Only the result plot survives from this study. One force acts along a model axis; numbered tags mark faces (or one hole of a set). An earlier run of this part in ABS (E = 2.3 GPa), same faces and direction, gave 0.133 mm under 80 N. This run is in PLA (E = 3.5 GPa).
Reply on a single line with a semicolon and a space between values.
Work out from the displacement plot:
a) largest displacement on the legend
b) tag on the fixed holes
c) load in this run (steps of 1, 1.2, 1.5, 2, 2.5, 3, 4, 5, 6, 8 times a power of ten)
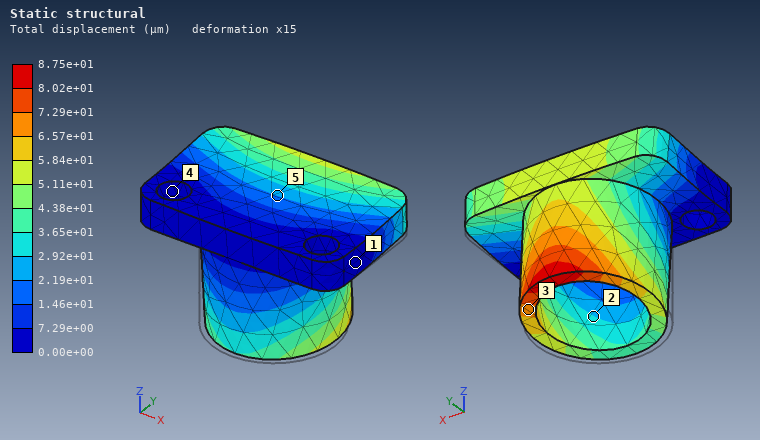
8.75e+01 µm; 4; 80 N
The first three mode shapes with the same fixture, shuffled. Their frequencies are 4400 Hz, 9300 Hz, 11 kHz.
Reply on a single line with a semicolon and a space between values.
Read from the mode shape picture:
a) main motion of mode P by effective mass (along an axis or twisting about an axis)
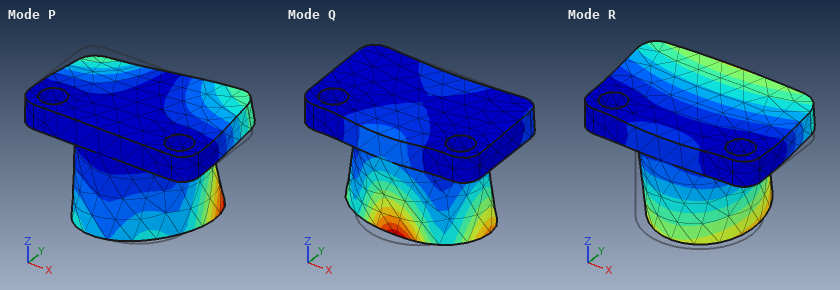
along X
